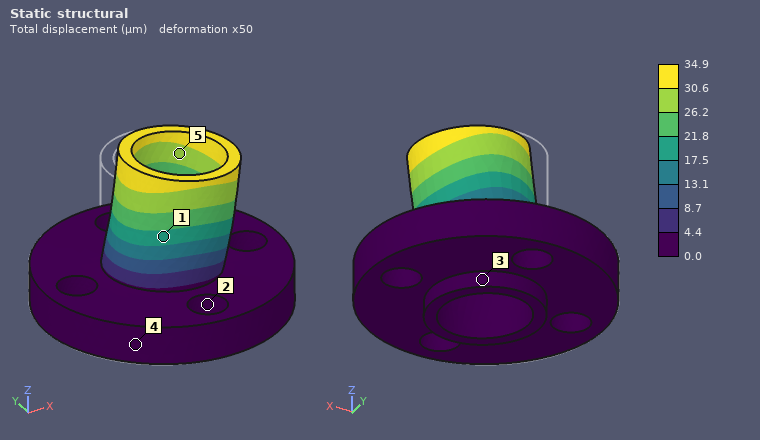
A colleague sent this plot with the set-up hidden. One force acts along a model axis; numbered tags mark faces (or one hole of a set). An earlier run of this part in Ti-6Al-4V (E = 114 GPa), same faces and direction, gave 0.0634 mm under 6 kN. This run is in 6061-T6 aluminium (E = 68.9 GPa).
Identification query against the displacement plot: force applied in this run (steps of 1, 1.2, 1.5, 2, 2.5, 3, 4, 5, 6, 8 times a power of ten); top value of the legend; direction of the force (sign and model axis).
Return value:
2 kN
34.9 µm
+X
